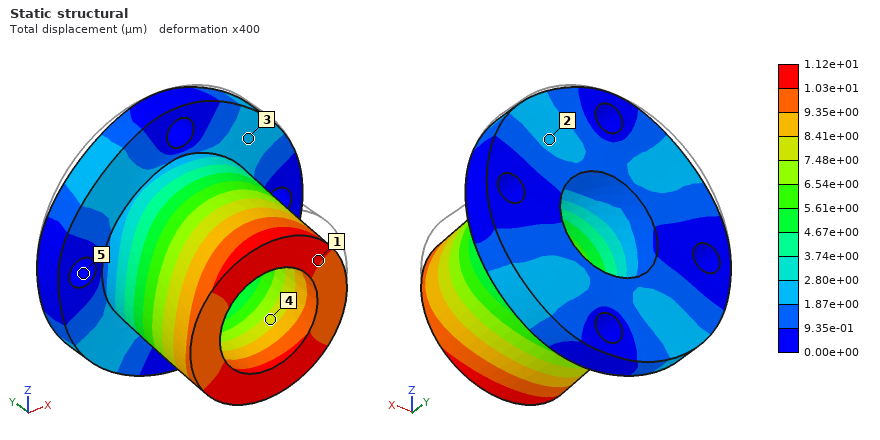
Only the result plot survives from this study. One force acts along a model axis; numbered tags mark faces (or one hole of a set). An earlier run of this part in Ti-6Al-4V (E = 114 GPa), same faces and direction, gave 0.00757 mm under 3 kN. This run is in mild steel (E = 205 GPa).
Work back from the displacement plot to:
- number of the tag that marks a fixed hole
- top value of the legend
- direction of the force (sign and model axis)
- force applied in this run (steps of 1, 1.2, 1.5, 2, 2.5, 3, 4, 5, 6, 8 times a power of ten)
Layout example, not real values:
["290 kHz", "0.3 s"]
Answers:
["5", "1.12e+01 µm", "-Z", "8 kN"]
